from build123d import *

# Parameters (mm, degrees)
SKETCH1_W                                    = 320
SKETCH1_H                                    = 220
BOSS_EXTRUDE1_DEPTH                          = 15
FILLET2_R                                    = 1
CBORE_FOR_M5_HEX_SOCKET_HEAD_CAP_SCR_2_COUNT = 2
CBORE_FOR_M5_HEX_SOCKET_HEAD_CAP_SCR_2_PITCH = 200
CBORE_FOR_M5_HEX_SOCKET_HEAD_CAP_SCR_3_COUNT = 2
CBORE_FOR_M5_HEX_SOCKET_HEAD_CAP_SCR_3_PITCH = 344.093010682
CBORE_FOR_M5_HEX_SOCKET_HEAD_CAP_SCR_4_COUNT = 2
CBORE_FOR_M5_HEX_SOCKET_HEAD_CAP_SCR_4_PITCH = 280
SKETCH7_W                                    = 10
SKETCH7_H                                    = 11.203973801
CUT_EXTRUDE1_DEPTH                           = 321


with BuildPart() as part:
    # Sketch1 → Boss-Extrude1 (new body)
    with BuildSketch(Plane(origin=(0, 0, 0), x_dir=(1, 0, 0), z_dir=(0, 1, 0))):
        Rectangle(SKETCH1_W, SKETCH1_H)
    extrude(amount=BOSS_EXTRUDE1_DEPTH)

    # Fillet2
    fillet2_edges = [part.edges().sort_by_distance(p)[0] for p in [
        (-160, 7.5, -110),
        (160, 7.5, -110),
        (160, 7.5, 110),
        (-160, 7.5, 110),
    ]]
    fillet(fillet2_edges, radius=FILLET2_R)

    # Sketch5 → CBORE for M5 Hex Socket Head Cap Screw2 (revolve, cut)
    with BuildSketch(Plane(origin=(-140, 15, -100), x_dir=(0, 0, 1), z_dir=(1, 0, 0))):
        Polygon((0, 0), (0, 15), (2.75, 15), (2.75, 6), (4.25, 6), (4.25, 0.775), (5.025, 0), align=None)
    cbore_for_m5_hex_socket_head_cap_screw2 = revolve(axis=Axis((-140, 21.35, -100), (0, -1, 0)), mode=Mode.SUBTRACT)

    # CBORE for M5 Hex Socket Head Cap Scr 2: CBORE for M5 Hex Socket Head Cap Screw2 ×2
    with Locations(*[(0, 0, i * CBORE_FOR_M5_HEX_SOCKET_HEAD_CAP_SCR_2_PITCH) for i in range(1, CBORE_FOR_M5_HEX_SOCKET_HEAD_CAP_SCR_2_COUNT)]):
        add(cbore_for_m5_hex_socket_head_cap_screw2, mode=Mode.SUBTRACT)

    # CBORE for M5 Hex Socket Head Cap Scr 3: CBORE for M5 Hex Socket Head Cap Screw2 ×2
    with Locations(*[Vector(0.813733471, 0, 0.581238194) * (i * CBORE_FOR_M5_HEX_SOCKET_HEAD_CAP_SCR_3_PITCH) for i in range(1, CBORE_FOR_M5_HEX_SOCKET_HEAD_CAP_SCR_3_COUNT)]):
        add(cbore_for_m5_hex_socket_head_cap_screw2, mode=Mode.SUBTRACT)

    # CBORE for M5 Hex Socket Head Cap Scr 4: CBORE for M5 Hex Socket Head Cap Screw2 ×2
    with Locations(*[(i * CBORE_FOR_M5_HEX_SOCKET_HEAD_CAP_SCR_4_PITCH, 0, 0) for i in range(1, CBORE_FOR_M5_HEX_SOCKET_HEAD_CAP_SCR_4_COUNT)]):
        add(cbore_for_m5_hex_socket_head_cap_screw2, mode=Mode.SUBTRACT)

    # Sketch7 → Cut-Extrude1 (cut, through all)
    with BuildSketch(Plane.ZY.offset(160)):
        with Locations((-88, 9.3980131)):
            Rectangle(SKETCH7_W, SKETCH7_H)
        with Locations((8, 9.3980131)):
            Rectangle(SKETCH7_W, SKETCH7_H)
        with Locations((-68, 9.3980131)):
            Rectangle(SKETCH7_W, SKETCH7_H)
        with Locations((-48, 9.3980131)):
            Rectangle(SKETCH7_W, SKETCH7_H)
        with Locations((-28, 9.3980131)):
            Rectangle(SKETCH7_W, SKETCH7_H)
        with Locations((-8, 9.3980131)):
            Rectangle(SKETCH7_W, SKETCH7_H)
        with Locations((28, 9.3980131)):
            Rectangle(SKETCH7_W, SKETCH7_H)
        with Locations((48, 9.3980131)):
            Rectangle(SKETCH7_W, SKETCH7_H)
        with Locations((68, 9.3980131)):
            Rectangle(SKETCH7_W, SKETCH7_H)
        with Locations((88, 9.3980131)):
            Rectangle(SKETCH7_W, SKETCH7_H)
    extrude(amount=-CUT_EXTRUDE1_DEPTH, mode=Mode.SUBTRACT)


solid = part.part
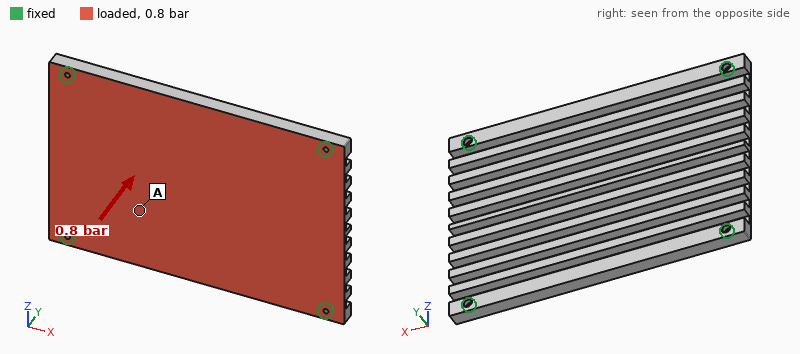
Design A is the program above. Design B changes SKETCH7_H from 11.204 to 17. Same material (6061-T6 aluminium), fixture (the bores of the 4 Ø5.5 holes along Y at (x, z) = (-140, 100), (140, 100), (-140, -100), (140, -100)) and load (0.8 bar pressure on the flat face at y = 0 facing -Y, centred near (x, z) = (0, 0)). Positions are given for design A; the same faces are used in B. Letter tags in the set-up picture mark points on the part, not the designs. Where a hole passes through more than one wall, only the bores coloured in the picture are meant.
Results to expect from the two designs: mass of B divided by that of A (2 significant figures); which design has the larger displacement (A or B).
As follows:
0.87
B
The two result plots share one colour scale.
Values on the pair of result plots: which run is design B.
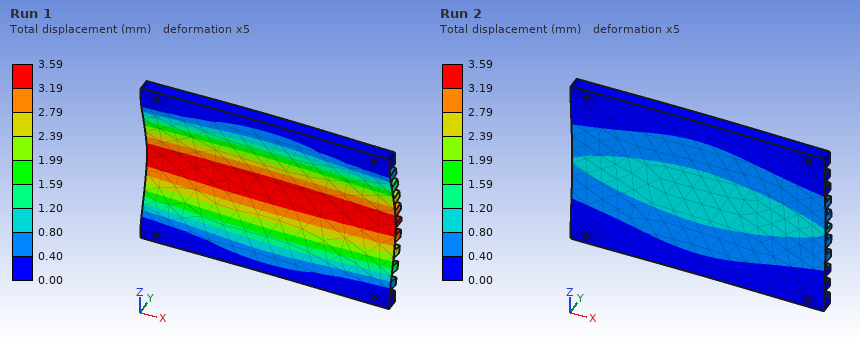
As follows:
Run 1
